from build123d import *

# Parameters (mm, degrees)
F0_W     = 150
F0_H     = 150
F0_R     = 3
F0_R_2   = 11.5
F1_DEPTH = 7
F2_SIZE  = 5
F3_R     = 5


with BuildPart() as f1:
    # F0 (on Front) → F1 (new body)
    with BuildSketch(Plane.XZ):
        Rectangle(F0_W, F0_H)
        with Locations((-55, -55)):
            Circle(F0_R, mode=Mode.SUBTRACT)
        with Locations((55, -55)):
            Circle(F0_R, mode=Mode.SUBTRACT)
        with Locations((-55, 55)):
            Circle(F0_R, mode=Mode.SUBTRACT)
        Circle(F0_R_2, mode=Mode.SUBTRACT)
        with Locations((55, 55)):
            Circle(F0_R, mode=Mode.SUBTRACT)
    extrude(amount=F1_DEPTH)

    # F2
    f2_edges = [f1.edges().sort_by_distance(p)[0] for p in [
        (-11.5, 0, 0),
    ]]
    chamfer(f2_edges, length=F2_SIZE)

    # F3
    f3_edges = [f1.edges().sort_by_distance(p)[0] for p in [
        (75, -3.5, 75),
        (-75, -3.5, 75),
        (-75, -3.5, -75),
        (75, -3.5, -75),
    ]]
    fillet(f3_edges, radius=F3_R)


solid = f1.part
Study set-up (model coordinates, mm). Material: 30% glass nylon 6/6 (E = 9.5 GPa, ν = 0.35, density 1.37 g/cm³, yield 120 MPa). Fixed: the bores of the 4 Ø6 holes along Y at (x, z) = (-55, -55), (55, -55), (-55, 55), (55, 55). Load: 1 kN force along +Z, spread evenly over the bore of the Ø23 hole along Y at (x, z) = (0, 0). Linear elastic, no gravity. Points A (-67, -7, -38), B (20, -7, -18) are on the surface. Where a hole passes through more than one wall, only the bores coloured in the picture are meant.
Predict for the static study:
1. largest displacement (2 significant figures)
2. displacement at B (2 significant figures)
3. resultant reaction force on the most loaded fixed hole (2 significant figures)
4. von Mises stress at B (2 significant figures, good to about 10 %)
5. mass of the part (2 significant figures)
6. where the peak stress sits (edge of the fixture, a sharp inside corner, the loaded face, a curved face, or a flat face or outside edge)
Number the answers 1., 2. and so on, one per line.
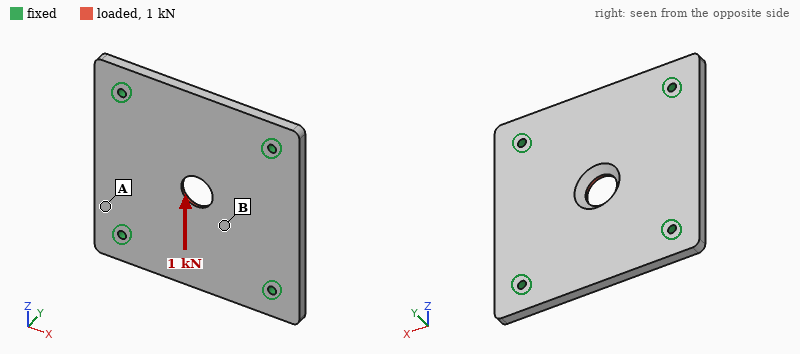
1. 18 µm
2. 11 µm
3. 270 N
4. 1.9 MPa
5. 210 g
6. the loaded face
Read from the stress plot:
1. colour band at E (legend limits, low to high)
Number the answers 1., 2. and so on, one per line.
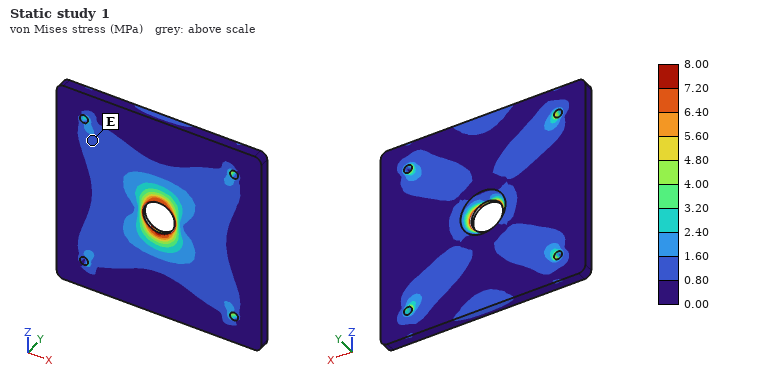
1. 0.80 to 1.60 MPa
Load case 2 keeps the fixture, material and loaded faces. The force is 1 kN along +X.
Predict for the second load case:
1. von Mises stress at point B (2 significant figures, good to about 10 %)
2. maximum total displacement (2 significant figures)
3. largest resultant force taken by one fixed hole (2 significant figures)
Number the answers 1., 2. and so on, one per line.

1. 2.0 MPa
2. 18 µm
3. 270 N
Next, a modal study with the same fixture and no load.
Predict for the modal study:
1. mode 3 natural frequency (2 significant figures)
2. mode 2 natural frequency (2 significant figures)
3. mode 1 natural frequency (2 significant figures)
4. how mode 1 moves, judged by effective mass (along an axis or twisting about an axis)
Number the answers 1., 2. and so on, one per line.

1. 1600 Hz
2. 1500 Hz
3. 1000 Hz
4. along Y
